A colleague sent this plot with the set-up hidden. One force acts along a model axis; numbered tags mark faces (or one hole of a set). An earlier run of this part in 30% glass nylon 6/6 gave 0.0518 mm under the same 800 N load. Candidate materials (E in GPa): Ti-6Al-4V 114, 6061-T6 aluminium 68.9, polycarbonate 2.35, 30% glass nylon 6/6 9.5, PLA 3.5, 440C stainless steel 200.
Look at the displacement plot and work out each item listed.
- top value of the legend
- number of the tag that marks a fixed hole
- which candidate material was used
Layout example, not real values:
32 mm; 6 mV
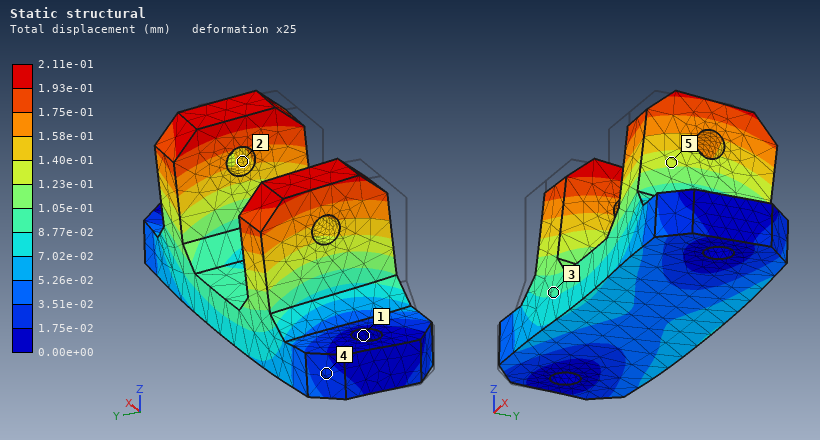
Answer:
2.11e-01 mm; 1; polycarbonate
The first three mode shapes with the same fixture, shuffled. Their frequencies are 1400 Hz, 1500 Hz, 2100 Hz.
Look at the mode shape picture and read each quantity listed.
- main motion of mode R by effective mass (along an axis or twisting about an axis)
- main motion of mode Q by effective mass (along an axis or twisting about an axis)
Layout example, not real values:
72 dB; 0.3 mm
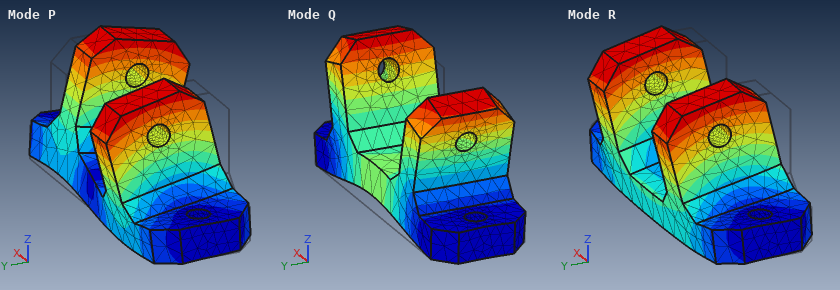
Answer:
along Y; along Z
